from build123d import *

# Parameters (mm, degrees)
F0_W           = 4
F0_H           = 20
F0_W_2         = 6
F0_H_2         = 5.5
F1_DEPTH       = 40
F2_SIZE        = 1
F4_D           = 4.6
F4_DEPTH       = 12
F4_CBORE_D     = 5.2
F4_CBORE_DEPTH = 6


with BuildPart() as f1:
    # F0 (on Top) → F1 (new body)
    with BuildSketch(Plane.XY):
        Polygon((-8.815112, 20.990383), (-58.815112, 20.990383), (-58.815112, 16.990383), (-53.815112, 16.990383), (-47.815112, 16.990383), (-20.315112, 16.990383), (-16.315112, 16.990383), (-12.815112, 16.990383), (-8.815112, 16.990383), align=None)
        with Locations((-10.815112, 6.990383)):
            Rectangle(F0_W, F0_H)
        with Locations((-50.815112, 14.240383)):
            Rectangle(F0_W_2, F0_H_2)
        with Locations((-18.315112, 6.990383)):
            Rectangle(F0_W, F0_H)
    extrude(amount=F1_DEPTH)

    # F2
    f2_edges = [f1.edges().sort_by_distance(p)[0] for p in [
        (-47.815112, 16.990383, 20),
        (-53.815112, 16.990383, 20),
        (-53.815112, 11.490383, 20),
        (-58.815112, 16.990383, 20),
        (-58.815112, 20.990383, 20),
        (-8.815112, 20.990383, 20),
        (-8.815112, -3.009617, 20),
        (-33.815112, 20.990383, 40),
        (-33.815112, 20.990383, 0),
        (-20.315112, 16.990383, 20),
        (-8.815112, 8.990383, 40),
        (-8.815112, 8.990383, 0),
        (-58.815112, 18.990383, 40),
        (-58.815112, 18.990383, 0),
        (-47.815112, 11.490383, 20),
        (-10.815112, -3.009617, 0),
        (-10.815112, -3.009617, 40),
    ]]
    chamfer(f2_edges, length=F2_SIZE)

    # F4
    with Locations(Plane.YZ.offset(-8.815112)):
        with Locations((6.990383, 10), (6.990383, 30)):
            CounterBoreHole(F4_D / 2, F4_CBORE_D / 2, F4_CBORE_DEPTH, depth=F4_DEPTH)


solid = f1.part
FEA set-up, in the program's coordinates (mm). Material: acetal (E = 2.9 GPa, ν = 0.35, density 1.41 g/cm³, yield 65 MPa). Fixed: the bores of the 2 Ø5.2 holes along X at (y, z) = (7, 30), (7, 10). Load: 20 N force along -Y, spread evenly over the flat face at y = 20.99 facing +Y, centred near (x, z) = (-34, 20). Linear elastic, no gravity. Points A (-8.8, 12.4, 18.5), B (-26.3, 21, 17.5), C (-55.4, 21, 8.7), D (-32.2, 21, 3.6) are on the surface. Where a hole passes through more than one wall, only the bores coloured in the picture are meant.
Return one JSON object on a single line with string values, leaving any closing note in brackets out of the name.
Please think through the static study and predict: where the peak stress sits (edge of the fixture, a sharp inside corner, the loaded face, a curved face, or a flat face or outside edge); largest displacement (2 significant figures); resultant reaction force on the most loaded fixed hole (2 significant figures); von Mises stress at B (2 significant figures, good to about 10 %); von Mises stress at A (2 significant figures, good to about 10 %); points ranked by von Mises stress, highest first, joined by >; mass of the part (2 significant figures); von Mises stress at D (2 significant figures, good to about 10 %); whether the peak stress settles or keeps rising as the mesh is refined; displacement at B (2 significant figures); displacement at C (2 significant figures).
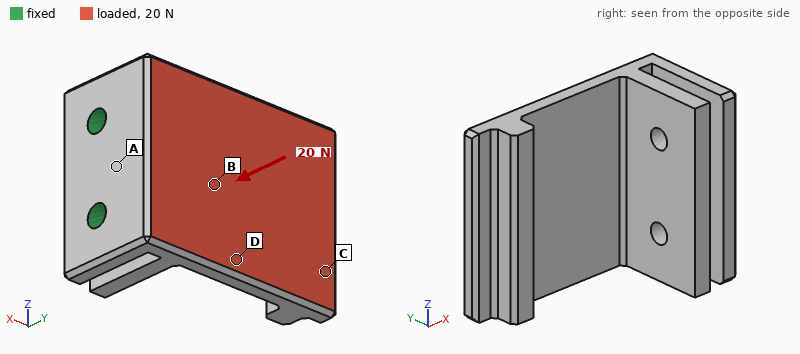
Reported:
{"where the peak stress sits": "edge of the fixture", "largest displacement": "0.69 mm", "resultant reaction force on the most loaded fixed hole": "10 N", "von Mises stress at B": "1.7 MPa", "von Mises stress at A": "3.3 MPa", "points ranked by von Mises stress, highest first, joined by >": "A > B > D > C", "mass of the part": "22 g", "von Mises stress at D": "1.3 MPa", "whether the peak stress settles or keeps rising as the mesh is refined": "keeps rising", "displacement at B": "0.18 mm", "displacement at C": "0.63 mm"}
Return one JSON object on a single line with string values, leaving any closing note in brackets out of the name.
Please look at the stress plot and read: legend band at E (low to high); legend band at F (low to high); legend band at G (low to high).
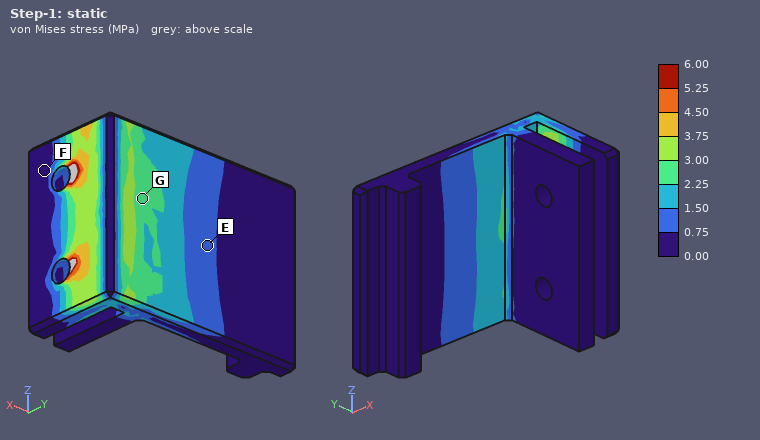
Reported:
{"legend band at E": "0.75 to 1.50 MPa", "legend band at F": "0.00 to 0.75 MPa", "legend band at G": "2.25 to 3.00 MPa"}
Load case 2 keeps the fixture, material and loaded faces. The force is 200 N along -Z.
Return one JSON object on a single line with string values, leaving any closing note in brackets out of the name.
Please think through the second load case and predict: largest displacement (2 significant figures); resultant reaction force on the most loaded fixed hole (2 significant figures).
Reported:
{"largest displacement": "0.75 mm", "resultant reaction force on the most loaded fixed hole": "240 N"}
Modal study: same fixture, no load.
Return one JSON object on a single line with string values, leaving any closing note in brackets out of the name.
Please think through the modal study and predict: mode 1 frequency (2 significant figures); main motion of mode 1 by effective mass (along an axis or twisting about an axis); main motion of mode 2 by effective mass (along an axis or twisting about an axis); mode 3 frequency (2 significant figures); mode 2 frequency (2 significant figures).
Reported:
{"mode 1 frequency": "260 Hz", "main motion of mode 1 by effective mass": "along Y", "main motion of mode 2 by effective mass": "along Z", "mode 3 frequency": "1100 Hz", "mode 2 frequency": "700 Hz"}
